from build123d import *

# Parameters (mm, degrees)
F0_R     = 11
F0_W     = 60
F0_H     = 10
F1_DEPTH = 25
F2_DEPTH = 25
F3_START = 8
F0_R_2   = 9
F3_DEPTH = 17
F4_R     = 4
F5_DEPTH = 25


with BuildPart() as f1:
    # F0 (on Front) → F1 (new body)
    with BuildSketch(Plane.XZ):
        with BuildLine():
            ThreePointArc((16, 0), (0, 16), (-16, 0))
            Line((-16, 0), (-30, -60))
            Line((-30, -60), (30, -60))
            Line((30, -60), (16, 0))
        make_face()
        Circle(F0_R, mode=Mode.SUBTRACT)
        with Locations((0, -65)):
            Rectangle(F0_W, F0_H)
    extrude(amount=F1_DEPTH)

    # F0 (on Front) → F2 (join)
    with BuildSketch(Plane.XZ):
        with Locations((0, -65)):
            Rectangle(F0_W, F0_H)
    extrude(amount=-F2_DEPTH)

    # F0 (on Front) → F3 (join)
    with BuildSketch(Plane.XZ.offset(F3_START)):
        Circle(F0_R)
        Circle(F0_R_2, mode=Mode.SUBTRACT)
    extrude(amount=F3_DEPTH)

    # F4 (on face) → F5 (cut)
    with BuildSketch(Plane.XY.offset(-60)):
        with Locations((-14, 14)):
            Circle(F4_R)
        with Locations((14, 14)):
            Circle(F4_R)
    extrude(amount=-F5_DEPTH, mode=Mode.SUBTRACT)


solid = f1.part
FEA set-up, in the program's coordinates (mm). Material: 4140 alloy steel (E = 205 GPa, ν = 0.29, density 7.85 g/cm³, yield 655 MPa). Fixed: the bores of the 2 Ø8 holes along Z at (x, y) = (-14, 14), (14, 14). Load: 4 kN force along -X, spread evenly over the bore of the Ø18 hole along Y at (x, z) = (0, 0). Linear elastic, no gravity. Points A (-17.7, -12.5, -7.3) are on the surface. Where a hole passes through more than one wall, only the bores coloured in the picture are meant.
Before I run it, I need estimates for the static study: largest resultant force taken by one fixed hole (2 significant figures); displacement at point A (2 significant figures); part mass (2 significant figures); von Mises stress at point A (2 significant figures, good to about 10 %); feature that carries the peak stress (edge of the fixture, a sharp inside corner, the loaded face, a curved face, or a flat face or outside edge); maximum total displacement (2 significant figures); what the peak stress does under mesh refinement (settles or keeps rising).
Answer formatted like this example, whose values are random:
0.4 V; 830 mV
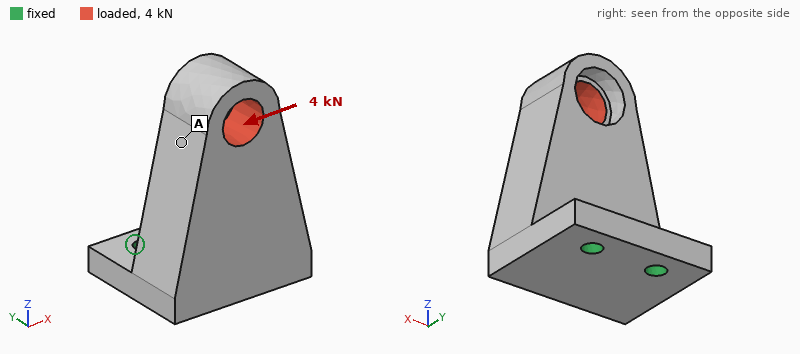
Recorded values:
7.9 kN; 63 µm; 790 g; 20 MPa; edge of the fixture; 88 µm; keeps rising
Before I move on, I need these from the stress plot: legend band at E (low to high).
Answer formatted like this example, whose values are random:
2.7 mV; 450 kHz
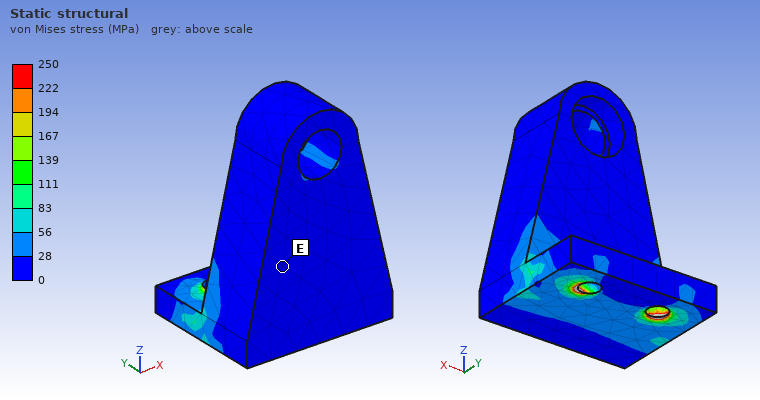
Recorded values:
0 to 28 MPa
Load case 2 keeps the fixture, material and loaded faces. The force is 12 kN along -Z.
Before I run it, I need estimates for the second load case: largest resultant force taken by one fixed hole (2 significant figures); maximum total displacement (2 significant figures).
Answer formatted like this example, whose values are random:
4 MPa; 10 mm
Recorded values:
6.0 kN; 0.40 mm
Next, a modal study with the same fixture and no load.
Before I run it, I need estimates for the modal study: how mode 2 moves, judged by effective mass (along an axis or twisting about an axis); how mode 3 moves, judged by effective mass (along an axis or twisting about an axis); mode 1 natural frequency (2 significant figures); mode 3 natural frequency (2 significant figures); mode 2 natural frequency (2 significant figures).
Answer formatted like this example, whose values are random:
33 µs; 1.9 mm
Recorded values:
along X; along Z; 1100 Hz; 6000 Hz; 2500 Hz
